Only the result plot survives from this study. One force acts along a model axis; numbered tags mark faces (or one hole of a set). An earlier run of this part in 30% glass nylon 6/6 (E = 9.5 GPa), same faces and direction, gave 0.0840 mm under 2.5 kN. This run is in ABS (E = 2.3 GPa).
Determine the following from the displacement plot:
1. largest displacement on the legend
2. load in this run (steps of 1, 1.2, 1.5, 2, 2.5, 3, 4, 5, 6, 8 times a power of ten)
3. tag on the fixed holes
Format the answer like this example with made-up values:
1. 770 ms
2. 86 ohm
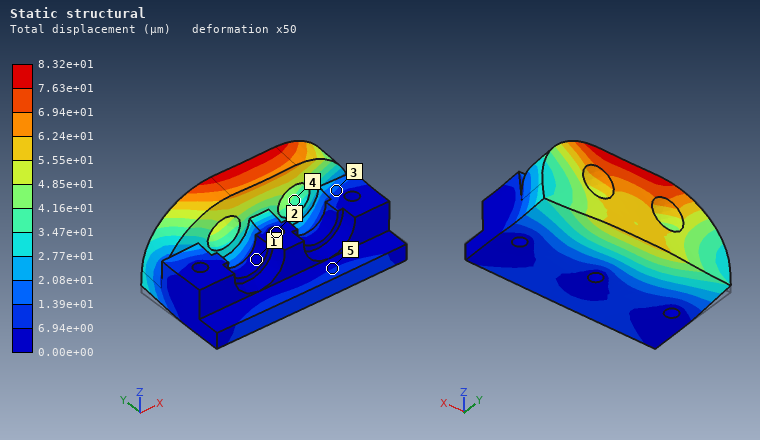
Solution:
1. 8.32e+01 µm
2. 600 N
3. 2
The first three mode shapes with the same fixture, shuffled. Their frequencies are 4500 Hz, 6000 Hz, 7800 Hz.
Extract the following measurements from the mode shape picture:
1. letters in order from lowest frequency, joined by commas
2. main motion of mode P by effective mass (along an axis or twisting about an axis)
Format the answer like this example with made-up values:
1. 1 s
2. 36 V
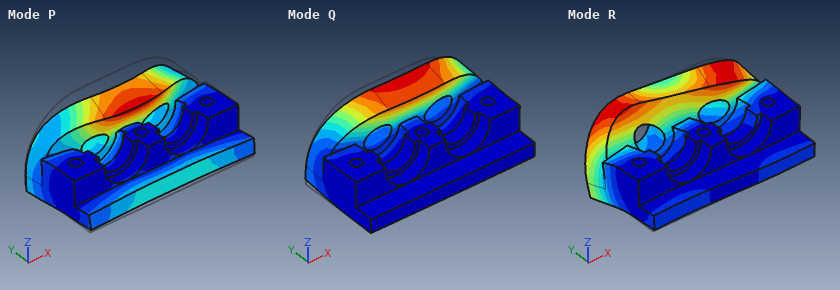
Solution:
1. Q, R, P
2. along Z
